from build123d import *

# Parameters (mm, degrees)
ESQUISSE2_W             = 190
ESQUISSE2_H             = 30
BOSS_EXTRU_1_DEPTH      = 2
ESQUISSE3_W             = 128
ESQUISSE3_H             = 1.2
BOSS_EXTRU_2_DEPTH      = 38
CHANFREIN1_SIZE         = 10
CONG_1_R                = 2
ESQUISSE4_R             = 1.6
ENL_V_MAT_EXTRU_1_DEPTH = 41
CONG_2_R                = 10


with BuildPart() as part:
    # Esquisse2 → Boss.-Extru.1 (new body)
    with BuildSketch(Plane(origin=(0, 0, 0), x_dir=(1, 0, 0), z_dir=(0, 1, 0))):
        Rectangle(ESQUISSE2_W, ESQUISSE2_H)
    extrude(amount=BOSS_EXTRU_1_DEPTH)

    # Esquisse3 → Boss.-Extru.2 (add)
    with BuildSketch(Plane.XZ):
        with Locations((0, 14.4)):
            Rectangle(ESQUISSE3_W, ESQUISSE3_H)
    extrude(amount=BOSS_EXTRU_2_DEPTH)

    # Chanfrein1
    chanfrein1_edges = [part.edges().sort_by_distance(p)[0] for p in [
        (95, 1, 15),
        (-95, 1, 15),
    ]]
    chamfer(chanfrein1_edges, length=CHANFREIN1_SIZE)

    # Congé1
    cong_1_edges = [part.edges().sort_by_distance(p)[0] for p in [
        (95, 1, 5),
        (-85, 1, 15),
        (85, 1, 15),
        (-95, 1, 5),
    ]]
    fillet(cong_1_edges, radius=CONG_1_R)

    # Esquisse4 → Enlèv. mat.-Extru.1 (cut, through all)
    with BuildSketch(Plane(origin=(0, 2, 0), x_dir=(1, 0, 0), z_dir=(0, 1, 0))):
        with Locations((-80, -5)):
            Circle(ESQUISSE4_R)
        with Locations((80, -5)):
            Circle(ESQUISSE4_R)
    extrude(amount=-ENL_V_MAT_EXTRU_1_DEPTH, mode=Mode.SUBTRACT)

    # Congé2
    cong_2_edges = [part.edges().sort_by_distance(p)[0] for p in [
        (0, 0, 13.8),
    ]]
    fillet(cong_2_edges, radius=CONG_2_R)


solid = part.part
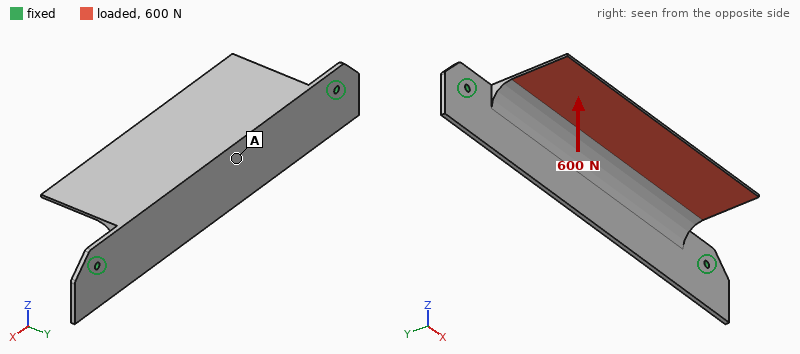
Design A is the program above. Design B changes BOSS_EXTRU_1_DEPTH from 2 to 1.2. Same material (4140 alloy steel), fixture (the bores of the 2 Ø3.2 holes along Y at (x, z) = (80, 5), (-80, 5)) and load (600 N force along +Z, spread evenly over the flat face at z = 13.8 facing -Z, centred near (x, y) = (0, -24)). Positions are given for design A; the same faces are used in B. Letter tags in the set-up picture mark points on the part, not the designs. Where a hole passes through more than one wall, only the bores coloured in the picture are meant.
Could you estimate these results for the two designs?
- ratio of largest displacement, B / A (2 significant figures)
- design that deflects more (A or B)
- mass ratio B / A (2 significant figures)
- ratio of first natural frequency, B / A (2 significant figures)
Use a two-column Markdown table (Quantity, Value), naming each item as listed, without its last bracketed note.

| Quantity | Value |
|---|---|
| ratio of largest displacement, B / A | 2.7 |
| design that deflects more | B |
| mass ratio B / A | 0.77 |
| ratio of first natural frequency, B / A | 0.58 |
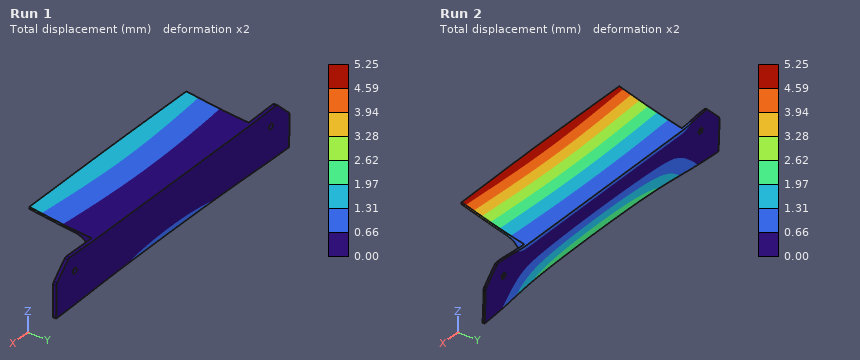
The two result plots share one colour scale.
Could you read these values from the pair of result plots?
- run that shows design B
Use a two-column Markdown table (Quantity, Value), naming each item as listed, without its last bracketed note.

| Quantity | Value |
|---|---|
| run that shows design B | Run 2 |
